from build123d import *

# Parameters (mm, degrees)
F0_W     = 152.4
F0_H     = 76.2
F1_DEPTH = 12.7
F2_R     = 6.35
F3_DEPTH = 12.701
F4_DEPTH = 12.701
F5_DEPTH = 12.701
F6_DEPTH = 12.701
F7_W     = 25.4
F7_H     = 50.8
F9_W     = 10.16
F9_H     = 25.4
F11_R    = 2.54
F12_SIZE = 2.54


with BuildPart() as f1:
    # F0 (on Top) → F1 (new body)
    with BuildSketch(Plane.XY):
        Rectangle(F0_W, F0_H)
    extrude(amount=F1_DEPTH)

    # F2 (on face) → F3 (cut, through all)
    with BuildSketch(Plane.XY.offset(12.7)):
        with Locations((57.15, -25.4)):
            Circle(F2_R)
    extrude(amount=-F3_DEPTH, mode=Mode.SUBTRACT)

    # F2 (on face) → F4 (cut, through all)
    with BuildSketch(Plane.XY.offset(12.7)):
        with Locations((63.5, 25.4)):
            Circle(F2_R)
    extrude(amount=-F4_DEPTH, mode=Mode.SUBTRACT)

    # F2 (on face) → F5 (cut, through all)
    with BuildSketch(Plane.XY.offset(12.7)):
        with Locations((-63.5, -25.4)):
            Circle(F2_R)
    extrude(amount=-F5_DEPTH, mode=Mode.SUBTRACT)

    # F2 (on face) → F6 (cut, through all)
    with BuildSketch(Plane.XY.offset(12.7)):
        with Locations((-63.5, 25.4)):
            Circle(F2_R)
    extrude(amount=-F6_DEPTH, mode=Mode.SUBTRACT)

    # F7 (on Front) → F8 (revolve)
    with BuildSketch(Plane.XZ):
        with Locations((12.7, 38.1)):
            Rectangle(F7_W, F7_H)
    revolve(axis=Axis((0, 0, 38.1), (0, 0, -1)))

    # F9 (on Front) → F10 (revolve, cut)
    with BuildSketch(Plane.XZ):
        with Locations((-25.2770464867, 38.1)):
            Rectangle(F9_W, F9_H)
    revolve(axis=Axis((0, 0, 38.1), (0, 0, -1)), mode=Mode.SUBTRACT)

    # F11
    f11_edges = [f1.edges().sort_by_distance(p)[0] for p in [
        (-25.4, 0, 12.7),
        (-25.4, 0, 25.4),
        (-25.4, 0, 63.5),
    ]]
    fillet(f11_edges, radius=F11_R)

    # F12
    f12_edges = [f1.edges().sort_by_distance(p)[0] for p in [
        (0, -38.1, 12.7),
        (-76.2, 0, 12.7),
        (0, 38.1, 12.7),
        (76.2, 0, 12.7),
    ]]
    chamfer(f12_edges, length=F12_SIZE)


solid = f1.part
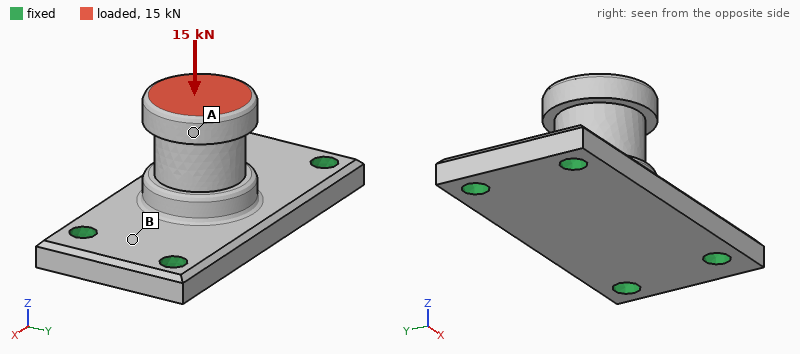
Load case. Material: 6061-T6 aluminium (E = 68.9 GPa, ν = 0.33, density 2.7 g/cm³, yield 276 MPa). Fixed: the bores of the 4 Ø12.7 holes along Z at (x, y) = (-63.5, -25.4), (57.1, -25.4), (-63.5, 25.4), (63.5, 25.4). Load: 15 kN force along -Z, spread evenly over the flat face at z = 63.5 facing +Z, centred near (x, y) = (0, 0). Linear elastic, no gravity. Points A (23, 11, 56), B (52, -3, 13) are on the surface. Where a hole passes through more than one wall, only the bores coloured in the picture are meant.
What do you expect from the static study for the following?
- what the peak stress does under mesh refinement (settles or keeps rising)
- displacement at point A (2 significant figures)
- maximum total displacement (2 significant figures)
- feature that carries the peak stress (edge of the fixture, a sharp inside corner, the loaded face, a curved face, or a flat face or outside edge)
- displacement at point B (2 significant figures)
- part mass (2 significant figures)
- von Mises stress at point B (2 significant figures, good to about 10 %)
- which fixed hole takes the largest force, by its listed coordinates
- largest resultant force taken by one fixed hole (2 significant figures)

keeps rising
90 µm
97 µm
edge of the fixture
16 µm
600 g
26 MPa
(57.1, -25.4)
4.8 kN
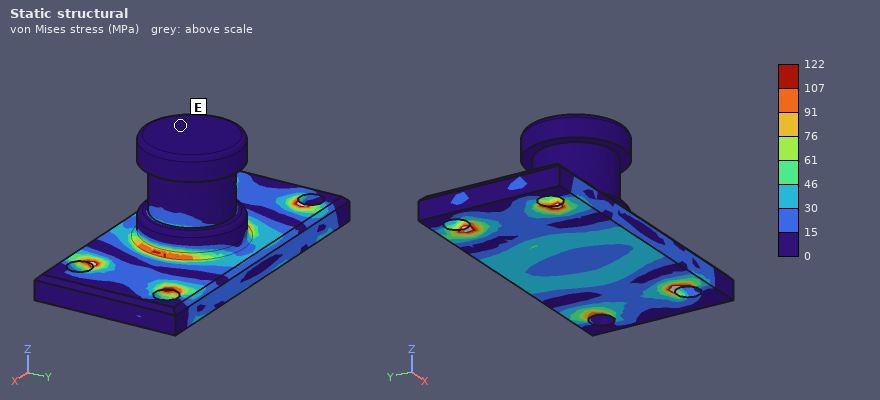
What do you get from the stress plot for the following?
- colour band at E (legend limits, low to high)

0 to 15 MPa
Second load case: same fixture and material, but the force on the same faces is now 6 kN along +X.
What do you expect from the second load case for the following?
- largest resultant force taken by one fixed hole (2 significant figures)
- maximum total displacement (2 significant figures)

2.7 kN
99 µm
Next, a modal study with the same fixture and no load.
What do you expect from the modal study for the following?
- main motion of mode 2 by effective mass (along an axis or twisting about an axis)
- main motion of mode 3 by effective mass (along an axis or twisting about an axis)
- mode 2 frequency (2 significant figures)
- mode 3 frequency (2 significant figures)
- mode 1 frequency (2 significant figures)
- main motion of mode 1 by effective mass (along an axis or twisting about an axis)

along Z
along X
3400 Hz
4300 Hz
2700 Hz
along Y
